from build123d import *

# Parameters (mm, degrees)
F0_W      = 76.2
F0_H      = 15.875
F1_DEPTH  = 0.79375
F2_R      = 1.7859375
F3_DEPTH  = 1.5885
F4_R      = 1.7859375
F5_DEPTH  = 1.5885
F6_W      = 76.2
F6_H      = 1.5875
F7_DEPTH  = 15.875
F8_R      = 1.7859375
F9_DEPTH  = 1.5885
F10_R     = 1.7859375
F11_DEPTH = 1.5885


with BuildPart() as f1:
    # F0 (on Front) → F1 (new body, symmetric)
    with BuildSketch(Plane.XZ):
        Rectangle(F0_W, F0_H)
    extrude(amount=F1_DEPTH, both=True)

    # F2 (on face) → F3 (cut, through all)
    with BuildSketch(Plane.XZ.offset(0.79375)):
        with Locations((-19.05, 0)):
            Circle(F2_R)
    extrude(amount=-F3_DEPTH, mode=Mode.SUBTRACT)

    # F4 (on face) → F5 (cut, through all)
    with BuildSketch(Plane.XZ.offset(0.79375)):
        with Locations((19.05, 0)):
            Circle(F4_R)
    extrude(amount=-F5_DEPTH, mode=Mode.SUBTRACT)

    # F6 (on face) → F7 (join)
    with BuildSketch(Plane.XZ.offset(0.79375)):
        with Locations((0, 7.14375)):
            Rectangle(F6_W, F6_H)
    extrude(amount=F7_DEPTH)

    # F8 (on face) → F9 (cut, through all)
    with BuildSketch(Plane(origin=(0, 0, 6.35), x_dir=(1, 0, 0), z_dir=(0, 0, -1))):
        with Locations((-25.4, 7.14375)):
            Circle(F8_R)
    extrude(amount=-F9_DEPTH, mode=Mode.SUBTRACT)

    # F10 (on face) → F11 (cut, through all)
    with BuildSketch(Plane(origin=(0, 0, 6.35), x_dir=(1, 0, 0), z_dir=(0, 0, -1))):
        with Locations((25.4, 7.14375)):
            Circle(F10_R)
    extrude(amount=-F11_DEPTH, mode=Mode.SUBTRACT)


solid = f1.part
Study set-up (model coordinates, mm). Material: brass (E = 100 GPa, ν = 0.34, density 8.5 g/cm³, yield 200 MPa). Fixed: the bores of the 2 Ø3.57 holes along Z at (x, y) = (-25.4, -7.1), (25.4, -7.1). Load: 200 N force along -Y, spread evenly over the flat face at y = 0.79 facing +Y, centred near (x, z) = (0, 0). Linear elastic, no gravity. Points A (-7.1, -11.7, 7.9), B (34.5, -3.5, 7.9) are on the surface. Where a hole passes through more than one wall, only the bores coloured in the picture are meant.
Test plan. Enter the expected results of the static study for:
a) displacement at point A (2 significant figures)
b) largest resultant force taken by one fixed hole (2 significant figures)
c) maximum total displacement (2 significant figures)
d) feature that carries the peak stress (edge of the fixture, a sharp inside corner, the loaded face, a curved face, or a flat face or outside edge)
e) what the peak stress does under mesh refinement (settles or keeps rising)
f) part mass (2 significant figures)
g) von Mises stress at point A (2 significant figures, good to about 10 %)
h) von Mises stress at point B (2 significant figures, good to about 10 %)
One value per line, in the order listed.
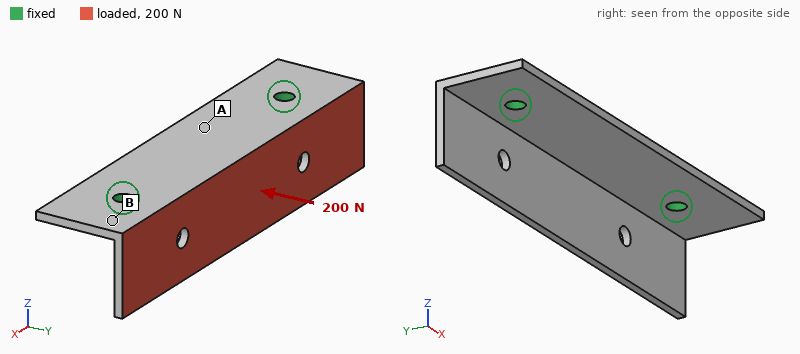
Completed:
0.030 mm
100 N
0.12 mm
edge of the fixture
keeps rising
32 g
16 MPa
36 MPa
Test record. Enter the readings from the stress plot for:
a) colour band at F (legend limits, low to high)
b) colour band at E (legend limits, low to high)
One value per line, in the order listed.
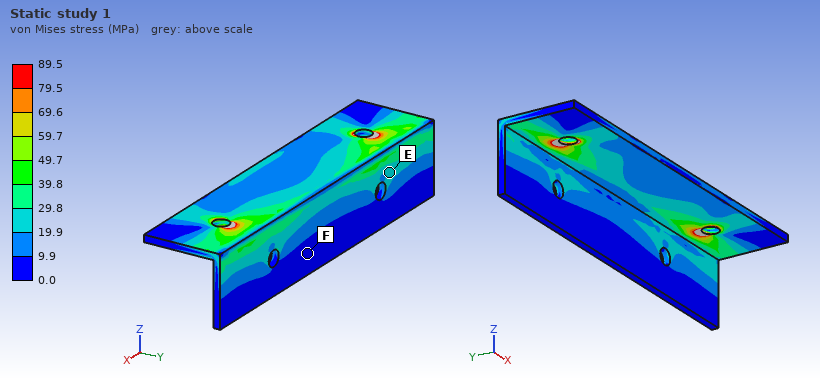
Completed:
0.0 to 9.9 MPa
19.9 to 29.8 MPa
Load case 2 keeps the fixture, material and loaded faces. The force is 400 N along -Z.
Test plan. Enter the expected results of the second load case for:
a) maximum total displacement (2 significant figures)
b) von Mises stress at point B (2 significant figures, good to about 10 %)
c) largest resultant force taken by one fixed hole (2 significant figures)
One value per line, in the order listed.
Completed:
0.12 mm
40 MPa
210 N
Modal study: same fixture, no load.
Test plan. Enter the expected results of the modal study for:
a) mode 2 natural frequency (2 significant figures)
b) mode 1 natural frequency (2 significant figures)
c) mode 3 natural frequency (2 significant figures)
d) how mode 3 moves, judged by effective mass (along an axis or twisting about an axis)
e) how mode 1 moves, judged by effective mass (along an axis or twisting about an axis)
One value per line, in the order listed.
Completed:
2600 Hz
1900 Hz
3200 Hz
along Z
along Y
